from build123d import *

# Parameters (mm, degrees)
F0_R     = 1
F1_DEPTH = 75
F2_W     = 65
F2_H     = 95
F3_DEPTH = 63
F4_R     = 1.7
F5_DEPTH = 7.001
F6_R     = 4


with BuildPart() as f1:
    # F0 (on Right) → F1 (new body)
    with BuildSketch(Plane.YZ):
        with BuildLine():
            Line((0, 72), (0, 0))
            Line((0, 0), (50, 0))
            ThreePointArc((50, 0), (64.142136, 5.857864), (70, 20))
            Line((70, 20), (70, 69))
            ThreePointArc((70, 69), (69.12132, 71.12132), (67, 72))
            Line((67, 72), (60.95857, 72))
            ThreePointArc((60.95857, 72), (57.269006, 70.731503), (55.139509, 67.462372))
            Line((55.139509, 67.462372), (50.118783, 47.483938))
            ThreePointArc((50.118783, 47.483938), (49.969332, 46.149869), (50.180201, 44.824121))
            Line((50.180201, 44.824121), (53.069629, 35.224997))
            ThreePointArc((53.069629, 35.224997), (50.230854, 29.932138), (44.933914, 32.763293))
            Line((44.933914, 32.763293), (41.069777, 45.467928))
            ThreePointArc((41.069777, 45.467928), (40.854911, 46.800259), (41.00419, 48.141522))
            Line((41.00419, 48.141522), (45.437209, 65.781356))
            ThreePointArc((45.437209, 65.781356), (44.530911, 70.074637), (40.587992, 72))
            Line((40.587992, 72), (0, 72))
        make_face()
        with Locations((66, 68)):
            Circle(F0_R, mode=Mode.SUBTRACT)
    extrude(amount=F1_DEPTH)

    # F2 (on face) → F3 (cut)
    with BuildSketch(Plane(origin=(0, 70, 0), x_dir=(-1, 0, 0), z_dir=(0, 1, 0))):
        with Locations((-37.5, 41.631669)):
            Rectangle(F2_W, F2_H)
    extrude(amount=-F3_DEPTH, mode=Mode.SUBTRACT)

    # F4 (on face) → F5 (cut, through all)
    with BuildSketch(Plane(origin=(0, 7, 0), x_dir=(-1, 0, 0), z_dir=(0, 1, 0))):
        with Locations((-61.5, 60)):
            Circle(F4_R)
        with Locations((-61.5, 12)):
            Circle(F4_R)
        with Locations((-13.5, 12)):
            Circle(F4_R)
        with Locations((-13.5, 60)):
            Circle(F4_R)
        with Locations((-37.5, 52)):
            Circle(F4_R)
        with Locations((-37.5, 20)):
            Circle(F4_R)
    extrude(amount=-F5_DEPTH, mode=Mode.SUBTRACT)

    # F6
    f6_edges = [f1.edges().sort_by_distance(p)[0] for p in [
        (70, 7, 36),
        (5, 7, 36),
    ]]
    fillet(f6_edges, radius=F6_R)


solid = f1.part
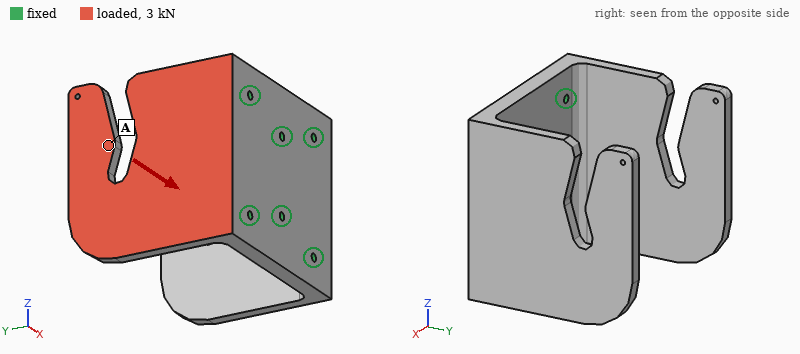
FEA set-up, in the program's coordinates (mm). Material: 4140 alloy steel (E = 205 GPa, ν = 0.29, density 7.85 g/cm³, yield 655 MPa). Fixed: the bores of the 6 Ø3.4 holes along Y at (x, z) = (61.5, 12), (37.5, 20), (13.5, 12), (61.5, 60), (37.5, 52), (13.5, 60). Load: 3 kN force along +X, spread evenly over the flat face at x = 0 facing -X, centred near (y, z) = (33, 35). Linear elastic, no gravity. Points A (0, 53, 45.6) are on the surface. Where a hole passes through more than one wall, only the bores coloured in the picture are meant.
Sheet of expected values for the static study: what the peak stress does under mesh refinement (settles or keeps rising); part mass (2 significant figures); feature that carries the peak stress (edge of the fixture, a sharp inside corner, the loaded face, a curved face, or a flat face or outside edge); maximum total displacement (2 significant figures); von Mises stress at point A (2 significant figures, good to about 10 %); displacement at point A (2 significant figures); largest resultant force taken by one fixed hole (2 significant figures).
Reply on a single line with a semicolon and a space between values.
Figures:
keeps rising; 620 g; edge of the fixture; 1.1 mm; 41 MPa; 0.63 mm; 1.4 kN
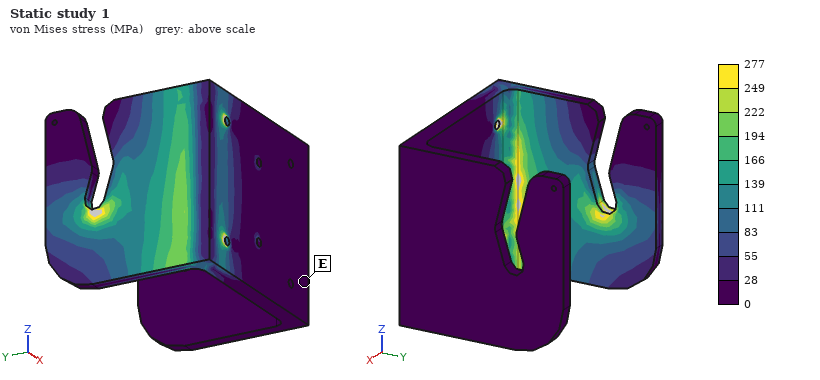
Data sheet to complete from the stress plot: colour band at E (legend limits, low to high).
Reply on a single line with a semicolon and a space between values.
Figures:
0 to 28 MPa
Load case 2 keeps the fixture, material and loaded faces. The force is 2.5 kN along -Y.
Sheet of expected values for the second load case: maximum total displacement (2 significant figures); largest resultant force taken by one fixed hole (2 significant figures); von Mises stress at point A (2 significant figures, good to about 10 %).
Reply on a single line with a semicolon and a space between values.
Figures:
0.11 mm; 1.6 kN; 11 MPa
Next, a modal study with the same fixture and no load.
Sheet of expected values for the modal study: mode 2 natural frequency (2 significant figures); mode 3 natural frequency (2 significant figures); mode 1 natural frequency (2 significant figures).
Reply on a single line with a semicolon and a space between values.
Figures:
830 Hz; 1600 Hz; 830 Hz
